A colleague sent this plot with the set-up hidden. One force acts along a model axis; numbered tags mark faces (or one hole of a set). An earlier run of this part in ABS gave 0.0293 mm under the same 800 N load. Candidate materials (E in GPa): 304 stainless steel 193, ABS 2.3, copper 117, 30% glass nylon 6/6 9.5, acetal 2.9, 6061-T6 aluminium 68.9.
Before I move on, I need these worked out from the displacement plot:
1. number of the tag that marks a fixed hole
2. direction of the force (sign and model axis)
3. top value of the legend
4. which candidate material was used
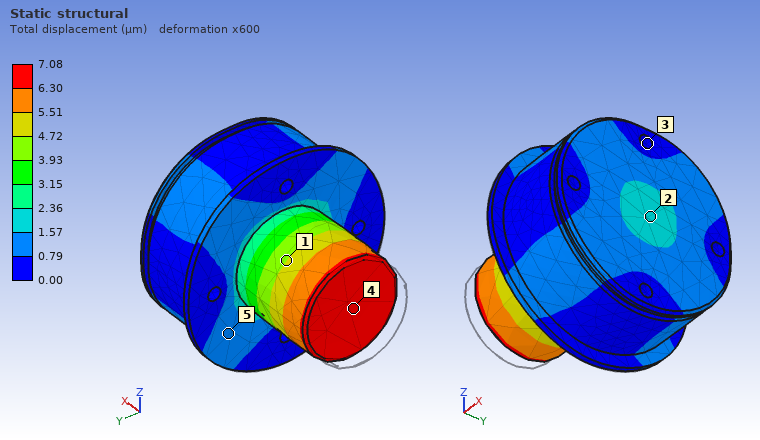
3
+X
7.08 µm
30% glass nylon 6/6
